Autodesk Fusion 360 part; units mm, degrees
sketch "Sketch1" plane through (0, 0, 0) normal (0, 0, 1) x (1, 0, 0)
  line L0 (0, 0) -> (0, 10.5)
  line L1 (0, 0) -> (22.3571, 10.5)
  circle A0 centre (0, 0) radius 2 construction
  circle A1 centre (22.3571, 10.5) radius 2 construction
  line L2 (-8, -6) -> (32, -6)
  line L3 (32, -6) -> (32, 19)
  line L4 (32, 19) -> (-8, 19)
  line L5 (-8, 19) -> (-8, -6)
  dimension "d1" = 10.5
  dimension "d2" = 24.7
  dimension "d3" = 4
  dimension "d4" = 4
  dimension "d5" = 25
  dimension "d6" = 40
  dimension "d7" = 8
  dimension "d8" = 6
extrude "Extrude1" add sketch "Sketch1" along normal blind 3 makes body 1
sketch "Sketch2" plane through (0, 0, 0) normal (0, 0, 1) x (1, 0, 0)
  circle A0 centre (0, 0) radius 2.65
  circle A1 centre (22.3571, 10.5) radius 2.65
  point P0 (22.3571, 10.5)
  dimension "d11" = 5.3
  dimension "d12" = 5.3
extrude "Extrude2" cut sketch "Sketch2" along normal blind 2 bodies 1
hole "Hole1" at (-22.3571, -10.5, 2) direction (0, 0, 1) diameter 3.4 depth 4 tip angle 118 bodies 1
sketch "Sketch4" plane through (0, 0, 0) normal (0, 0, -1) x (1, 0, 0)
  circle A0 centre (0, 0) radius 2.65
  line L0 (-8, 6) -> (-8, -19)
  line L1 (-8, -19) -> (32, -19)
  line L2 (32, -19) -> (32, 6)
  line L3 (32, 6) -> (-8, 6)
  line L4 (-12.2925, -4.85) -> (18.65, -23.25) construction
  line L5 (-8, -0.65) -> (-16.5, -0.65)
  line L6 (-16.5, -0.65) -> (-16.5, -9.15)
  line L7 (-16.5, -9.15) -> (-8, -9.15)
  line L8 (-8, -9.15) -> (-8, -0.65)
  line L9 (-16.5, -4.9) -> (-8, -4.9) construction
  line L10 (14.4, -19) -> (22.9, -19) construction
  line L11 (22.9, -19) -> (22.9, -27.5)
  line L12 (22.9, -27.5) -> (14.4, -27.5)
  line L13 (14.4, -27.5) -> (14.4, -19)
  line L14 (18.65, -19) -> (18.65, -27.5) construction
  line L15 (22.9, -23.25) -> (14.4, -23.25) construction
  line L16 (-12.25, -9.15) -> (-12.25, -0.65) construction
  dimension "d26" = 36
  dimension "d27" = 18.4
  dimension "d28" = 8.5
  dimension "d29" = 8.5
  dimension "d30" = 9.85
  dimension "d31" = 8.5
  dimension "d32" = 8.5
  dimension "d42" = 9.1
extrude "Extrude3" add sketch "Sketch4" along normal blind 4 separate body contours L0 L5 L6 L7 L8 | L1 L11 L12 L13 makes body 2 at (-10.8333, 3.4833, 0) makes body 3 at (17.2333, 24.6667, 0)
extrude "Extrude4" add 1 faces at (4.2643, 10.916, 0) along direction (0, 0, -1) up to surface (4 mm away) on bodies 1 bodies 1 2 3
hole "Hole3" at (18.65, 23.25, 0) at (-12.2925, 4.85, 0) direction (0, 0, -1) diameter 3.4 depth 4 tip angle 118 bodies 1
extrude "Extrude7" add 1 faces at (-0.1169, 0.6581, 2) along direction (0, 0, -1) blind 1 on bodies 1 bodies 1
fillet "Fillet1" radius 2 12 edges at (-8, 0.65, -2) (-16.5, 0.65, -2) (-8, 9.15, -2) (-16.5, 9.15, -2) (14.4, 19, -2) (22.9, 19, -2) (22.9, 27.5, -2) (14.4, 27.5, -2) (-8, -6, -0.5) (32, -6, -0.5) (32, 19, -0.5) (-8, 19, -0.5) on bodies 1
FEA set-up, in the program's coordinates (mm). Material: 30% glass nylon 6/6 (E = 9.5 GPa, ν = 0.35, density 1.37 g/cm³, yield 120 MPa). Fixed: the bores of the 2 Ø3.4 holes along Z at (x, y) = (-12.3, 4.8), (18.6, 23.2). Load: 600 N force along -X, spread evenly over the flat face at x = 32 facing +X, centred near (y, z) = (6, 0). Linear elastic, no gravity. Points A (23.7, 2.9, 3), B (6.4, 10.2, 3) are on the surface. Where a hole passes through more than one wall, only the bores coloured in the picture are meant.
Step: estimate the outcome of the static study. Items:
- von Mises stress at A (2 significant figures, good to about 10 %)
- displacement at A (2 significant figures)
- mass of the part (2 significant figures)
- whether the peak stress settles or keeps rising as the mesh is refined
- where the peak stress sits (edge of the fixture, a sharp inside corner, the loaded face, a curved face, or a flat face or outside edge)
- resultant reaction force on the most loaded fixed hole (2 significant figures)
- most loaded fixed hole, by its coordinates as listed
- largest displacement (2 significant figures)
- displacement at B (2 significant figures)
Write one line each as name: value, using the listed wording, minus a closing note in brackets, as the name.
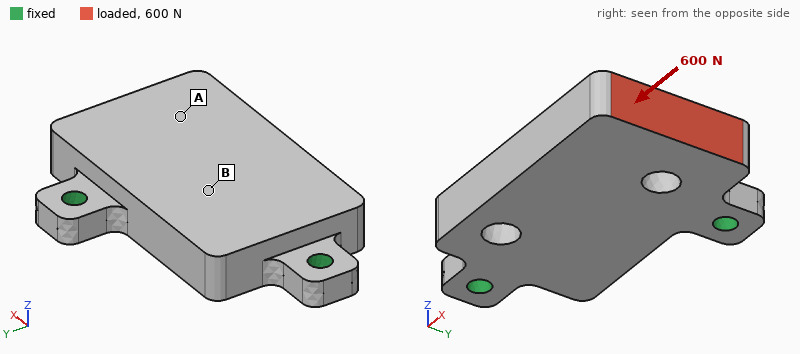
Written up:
von Mises stress at A: 4.0 MPa
displacement at A: 43 µm
mass of the part: 9.9 g
whether the peak stress settles or keeps rising as the mesh is refined: keeps rising
where the peak stress sits: edge of the fixture
resultant reaction force on the most loaded fixed hole: 420 N
most loaded fixed hole, by its coordinates as listed: (-12.3, 4.8)
largest displacement: 63 µm
displacement at B: 22 µm
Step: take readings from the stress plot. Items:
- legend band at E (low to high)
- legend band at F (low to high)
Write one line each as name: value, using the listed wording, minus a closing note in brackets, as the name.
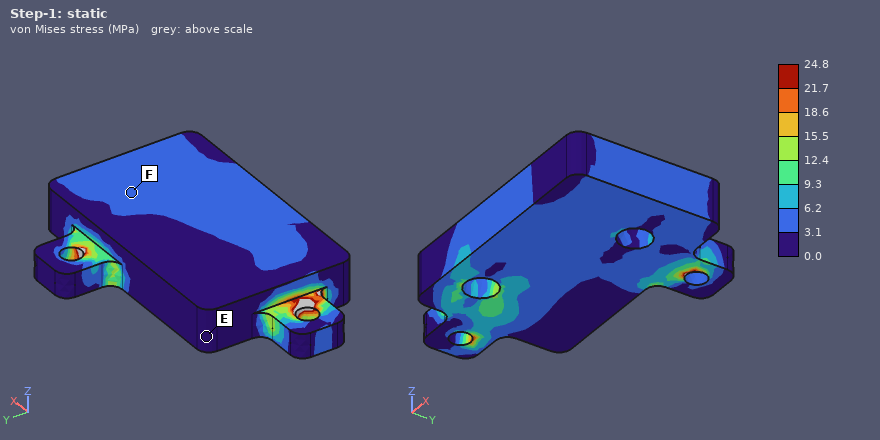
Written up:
legend band at E: 0.0 to 3.1 MPa
legend band at F: 3.1 to 6.2 MPa
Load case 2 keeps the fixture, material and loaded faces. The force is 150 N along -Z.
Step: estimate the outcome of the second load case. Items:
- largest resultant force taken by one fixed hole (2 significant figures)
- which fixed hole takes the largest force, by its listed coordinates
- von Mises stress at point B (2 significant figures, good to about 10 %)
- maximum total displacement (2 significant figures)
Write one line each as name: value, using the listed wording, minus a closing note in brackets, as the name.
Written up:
largest resultant force taken by one fixed hole: 170 N
which fixed hole takes the largest force, by its listed coordinates: (18.6, 23.2)
von Mises stress at point B: 7.3 MPa
maximum total displacement: 0.49 mm
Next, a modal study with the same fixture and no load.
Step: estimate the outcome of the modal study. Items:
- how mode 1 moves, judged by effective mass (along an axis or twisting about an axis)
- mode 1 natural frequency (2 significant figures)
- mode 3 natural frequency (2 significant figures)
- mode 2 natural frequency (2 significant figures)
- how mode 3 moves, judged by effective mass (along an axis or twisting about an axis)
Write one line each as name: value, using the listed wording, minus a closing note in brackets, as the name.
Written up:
how mode 1 moves, judged by effective mass: along Z
mode 1 natural frequency: 1800 Hz
mode 3 natural frequency: 8200 Hz
mode 2 natural frequency: 6800 Hz
how mode 3 moves, judged by effective mass: along Z
